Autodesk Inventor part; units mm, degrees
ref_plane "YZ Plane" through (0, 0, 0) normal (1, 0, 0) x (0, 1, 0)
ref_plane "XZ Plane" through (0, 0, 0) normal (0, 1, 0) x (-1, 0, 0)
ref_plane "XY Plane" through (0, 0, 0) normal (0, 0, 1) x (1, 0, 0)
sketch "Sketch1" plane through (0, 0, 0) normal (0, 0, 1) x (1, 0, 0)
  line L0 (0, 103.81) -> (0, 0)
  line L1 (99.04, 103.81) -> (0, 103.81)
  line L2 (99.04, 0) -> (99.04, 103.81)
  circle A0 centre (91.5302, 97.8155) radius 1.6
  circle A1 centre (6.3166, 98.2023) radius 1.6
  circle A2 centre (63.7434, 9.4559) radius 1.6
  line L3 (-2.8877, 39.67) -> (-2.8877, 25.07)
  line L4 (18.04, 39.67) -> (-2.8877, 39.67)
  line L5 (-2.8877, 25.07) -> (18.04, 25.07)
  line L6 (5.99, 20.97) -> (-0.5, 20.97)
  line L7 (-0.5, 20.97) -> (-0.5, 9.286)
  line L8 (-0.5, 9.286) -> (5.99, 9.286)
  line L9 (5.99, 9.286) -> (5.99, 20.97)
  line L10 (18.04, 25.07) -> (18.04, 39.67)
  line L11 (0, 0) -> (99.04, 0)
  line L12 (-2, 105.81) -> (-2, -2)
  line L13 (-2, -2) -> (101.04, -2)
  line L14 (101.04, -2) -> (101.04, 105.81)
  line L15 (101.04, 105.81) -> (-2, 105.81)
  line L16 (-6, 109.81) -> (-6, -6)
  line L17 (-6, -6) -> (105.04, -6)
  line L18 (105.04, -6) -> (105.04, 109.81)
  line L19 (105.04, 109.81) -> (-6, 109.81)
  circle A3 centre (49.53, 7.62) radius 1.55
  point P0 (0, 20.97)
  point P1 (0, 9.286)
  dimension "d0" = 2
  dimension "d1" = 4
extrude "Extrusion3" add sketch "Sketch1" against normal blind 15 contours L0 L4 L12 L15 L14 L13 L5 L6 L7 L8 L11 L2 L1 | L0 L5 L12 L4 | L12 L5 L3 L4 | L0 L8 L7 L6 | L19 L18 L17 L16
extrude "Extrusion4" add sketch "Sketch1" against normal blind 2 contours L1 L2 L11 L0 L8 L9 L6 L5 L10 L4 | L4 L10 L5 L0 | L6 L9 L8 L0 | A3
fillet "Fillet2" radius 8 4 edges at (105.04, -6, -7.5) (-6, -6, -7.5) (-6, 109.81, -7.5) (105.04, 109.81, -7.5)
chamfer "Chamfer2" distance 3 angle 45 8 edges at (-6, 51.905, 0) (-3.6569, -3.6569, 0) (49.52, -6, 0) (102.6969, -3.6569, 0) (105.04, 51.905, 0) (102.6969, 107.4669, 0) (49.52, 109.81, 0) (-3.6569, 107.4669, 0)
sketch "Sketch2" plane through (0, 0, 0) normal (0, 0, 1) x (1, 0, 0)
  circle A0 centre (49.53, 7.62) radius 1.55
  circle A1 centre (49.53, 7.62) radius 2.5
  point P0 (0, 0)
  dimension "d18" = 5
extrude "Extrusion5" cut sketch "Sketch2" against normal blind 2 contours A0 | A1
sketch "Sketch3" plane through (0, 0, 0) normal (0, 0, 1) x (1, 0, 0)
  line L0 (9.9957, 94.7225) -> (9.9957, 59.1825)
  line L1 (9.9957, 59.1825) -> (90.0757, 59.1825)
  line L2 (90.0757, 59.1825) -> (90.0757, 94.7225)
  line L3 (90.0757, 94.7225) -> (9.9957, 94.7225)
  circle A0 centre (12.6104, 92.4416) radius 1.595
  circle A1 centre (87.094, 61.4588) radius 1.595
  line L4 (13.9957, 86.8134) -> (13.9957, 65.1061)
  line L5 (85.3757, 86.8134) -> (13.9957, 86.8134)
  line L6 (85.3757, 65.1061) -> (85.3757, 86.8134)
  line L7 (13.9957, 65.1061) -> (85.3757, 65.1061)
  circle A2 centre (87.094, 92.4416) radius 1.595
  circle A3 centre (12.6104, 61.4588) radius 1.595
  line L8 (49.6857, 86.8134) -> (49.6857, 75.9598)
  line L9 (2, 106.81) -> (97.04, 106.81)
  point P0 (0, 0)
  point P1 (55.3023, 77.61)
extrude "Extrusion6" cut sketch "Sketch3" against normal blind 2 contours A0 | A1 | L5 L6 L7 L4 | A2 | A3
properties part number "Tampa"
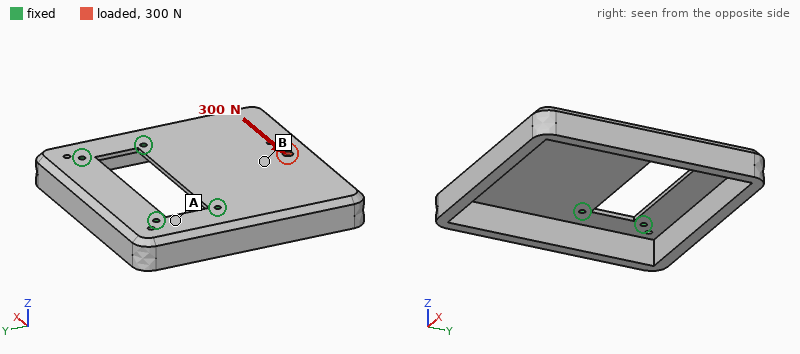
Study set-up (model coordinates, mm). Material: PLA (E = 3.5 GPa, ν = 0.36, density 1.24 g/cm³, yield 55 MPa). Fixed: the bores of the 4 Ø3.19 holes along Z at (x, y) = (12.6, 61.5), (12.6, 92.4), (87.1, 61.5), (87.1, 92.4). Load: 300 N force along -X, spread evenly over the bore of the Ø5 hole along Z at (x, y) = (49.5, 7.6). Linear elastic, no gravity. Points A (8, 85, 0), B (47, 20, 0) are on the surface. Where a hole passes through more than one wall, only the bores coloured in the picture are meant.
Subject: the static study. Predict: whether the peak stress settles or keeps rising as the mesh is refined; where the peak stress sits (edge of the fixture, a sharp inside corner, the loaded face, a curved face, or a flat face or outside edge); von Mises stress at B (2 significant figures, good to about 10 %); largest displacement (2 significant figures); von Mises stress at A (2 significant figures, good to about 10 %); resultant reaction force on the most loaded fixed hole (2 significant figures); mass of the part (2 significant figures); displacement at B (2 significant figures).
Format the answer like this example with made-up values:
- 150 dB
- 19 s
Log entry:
- keeps rising
- edge of the fixture
- 3.6 MPa
- 0.19 mm
- 2.0 MPa
- 220 N
- 66 g
- 0.088 mm
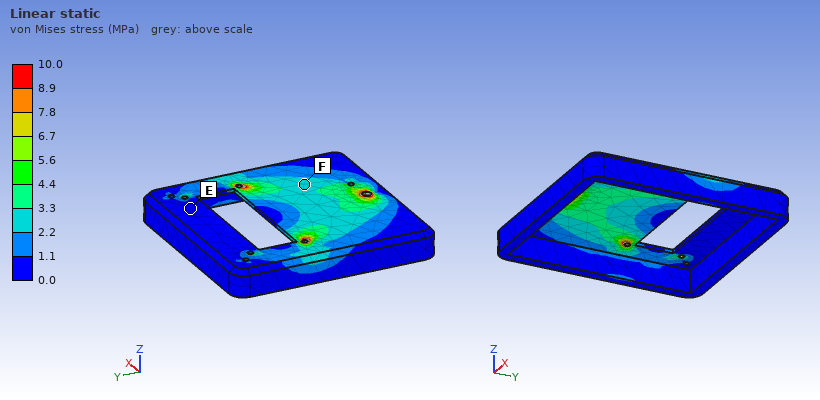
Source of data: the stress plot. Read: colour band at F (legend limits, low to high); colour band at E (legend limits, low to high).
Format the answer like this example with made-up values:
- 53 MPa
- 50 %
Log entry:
- 2.2 to 3.3 MPa
- 0.0 to 1.1 MPa
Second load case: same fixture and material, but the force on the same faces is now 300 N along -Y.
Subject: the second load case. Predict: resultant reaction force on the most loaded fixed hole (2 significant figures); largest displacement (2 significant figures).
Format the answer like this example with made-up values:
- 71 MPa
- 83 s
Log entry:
- 150 N
- 89 µm
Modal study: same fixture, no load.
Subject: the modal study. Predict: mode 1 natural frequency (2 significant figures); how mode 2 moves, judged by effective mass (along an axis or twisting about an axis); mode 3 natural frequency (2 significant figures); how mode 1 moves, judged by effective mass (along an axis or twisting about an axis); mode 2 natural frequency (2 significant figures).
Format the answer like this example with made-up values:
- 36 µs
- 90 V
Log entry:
- 210 Hz
- twisting about Y
- 620 Hz
- along Z
- 310 Hz
